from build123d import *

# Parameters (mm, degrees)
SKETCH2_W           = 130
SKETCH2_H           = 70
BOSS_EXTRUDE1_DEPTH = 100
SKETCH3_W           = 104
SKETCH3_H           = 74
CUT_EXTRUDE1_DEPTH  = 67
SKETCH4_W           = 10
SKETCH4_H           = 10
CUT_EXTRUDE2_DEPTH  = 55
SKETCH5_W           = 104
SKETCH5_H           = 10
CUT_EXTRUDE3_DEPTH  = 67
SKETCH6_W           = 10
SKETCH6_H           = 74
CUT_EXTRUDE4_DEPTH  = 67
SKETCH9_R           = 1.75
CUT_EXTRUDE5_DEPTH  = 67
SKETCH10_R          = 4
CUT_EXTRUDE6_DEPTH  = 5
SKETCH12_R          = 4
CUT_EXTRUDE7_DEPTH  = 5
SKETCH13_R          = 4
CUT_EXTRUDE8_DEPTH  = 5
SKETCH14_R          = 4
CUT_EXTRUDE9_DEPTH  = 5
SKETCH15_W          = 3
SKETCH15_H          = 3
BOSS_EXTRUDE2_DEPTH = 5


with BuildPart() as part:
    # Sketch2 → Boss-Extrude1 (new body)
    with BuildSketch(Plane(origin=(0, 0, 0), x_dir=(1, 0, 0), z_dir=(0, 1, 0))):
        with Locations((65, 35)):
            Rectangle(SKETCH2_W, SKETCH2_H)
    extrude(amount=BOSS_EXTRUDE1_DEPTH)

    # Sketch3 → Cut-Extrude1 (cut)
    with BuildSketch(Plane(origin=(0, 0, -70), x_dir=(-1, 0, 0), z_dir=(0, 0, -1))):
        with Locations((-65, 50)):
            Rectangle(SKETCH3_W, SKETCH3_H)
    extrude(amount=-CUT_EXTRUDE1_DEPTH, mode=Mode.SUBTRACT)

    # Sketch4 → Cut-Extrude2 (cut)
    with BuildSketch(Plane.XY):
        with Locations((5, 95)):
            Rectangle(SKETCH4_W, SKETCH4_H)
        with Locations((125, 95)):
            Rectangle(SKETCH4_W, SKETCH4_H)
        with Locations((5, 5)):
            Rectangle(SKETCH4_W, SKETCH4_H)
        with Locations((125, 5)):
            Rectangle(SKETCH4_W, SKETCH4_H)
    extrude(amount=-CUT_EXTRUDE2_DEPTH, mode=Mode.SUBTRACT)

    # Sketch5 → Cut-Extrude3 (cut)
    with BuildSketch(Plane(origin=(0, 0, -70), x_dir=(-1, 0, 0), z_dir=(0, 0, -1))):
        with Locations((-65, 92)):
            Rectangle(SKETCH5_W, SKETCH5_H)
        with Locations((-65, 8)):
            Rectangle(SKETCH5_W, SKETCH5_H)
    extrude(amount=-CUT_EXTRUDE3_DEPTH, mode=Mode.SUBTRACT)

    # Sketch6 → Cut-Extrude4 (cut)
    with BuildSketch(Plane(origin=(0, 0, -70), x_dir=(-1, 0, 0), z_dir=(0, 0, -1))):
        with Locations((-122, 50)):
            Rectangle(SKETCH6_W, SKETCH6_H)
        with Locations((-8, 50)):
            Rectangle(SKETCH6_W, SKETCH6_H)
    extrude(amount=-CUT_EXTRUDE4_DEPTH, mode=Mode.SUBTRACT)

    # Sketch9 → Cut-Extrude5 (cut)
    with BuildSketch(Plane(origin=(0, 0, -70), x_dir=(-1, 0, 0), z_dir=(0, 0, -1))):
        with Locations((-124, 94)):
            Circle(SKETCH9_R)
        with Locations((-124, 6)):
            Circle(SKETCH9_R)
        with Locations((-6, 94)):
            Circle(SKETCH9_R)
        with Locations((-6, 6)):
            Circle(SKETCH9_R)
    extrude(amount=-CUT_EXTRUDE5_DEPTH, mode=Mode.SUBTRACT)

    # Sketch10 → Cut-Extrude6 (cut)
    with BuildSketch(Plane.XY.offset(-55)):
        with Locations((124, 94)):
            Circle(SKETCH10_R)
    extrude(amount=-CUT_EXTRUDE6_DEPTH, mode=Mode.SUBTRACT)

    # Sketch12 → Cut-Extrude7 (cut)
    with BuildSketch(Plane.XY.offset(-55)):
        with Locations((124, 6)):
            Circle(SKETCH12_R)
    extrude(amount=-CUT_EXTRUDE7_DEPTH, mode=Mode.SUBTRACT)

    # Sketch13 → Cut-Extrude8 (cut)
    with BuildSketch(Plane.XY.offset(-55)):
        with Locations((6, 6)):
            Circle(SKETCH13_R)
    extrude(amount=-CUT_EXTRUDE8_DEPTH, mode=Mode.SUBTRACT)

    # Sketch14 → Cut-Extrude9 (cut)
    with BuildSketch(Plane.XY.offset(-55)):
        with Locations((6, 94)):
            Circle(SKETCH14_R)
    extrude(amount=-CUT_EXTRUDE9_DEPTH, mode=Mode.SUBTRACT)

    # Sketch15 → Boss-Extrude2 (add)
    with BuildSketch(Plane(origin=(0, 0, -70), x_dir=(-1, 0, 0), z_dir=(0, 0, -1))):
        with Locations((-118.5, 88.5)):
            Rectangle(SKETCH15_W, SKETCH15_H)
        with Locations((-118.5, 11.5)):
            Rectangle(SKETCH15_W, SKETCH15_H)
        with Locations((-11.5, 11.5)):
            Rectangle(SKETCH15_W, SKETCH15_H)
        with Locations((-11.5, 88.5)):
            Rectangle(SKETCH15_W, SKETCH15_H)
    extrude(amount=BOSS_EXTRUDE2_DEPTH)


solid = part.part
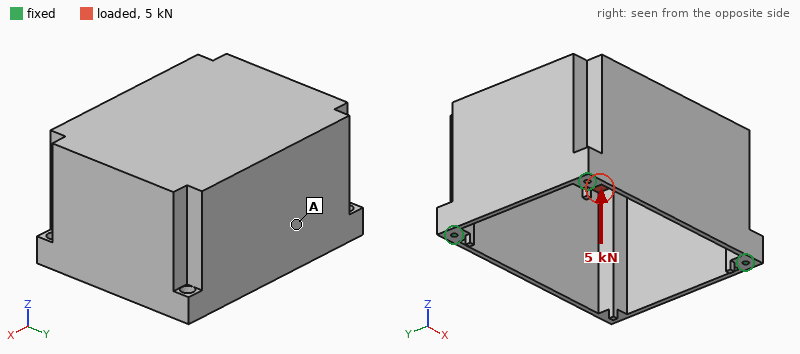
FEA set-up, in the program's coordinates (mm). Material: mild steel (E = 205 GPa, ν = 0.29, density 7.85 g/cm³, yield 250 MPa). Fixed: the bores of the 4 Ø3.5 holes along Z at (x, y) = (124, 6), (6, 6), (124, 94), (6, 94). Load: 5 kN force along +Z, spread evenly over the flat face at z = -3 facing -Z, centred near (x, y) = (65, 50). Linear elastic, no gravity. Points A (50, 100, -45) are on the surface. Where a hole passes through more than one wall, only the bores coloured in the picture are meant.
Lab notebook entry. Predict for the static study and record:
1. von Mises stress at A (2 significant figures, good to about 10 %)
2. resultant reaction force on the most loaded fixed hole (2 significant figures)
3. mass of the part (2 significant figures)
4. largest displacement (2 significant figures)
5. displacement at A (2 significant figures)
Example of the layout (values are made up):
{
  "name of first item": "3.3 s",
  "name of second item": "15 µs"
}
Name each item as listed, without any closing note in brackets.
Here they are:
{
  "von Mises stress at A": "17 MPa",
  "resultant reaction force on the most loaded fixed hole": "1.3 kN",
  "mass of the part": "1.0 kg",
  "largest displacement": "0.23 mm",
  "displacement at A": "0.040 mm"
}
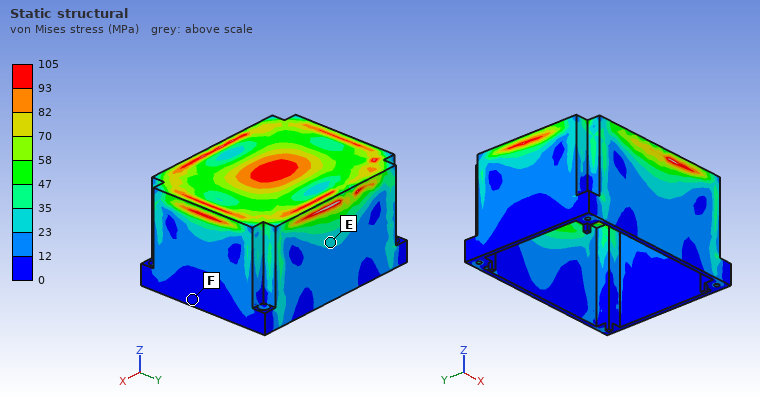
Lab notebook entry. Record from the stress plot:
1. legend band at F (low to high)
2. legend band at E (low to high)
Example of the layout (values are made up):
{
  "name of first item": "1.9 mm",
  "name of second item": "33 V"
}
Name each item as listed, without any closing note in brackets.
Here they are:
{
  "legend band at F": "0 to 12 MPa",
  "legend band at E": "23 to 35 MPa"
}
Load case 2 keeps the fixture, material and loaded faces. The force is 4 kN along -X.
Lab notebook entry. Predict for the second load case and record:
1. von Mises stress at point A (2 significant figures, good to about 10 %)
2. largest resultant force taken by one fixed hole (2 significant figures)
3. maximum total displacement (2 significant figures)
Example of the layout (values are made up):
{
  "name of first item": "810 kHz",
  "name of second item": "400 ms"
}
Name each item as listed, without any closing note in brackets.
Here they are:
{
  "von Mises stress at point A": "9.4 MPa",
  "largest resultant force taken by one fixed hole": "1.4 kN",
  "maximum total displacement": "9.8 µm"
}
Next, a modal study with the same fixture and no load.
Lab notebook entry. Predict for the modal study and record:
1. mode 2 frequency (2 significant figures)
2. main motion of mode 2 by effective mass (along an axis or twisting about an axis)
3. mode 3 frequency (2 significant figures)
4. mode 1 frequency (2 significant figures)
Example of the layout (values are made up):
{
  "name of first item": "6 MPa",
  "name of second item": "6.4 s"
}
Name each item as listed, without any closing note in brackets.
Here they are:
{
  "mode 2 frequency": "1600 Hz",
  "main motion of mode 2 by effective mass": "along Y",
  "mode 3 frequency": "1900 Hz",
  "mode 1 frequency": "1500 Hz"
}
